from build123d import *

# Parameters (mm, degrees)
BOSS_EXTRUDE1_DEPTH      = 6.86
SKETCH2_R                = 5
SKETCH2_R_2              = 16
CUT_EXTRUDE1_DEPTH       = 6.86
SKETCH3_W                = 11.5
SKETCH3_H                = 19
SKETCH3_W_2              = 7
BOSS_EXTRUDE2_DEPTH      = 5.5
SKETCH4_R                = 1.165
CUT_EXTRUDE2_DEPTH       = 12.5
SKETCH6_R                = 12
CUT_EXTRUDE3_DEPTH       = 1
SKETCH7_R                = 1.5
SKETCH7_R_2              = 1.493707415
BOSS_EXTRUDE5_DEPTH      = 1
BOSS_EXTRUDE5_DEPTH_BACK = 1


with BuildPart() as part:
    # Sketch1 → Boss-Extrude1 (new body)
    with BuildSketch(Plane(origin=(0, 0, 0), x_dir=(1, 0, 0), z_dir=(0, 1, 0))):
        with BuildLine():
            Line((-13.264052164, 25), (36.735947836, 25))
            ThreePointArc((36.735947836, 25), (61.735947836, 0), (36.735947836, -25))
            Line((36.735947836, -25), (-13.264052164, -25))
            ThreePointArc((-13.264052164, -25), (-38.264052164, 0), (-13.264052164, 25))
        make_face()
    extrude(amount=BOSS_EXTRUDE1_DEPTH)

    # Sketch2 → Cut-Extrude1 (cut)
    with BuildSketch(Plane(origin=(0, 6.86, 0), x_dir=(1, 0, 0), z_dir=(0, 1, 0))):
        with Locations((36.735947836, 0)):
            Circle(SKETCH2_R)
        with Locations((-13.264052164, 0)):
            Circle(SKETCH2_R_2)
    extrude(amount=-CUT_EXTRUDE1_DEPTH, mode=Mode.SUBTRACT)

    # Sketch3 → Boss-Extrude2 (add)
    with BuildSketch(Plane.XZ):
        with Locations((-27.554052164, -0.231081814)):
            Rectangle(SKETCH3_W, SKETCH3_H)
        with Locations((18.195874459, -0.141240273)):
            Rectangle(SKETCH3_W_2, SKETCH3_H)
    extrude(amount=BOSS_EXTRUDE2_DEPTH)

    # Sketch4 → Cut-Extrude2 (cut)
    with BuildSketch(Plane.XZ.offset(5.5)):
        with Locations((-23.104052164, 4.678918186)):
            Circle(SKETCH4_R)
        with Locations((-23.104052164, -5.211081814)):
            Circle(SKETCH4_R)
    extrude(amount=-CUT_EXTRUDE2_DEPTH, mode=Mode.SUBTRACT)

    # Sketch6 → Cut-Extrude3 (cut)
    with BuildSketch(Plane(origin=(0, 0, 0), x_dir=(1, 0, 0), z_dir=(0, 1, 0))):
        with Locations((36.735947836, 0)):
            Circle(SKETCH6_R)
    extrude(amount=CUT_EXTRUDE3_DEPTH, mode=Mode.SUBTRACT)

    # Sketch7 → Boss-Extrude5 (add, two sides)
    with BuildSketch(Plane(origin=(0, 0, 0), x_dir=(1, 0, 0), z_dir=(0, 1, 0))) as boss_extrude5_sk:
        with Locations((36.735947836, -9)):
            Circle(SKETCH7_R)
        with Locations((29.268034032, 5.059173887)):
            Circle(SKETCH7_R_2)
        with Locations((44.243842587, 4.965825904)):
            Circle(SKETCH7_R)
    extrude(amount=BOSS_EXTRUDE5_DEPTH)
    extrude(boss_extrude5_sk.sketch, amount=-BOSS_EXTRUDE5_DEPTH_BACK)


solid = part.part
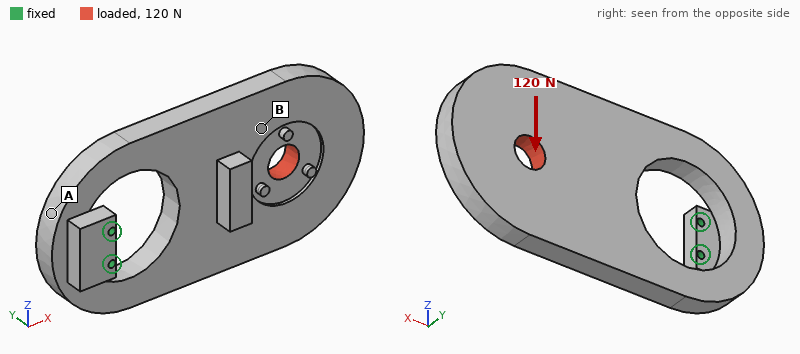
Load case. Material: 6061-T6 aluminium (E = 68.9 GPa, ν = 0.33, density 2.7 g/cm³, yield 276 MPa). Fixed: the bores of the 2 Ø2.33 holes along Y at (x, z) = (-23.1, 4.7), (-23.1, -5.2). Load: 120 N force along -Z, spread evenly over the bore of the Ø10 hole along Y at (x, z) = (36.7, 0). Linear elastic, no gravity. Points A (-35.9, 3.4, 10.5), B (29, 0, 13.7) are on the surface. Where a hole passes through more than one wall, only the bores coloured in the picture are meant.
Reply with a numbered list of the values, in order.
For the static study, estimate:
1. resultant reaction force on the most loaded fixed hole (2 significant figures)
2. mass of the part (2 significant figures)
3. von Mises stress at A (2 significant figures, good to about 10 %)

1. 640 N
2. 71 g
3. 18 MPa
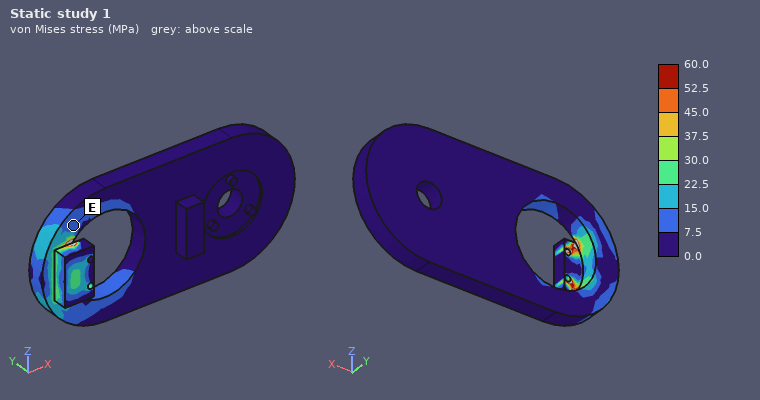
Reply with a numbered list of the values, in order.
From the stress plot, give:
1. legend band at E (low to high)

1. 7.5 to 15.0 MPa
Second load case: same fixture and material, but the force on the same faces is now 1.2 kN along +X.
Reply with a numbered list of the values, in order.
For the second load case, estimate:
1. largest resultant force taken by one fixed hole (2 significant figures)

1. 650 N
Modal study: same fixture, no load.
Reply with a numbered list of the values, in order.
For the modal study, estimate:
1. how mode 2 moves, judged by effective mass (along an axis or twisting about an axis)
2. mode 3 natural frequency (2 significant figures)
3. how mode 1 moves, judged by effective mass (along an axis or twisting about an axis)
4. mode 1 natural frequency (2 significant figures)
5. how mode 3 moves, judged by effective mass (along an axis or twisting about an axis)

1. along Z
2. 1700 Hz
3. along Y
4. 320 Hz
5. twisting about X
